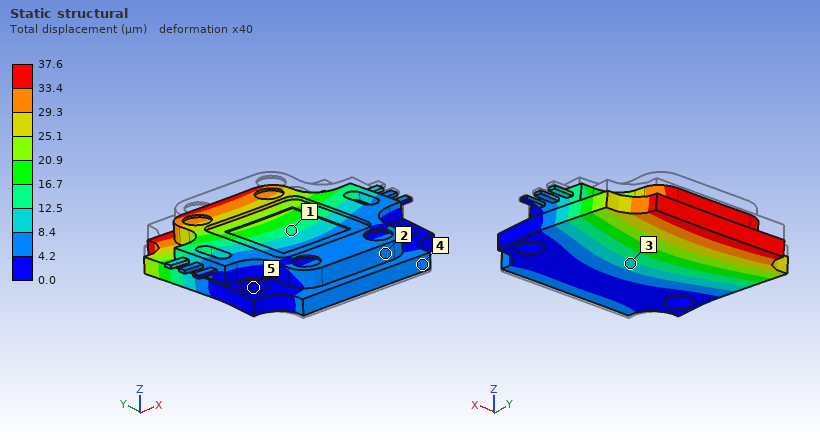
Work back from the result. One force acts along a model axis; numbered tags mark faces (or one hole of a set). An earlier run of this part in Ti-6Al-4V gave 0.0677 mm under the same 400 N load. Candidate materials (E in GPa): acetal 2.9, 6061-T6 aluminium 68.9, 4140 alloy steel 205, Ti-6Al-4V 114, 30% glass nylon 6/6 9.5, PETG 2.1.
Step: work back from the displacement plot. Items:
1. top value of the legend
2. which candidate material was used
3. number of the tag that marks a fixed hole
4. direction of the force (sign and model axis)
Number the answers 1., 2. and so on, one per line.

1. 37.6 µm
2. 4140 alloy steel
3. 5
4. -Z
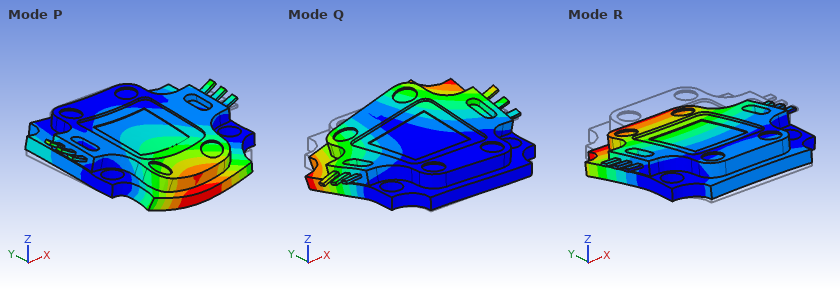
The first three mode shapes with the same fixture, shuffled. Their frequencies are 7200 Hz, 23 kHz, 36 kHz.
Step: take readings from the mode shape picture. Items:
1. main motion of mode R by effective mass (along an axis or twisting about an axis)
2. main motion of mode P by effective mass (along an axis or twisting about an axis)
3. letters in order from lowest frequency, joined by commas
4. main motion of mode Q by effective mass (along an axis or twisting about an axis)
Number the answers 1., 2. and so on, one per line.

1. along Z
2. along Z
3. R, Q, P
4. twisting about Y
